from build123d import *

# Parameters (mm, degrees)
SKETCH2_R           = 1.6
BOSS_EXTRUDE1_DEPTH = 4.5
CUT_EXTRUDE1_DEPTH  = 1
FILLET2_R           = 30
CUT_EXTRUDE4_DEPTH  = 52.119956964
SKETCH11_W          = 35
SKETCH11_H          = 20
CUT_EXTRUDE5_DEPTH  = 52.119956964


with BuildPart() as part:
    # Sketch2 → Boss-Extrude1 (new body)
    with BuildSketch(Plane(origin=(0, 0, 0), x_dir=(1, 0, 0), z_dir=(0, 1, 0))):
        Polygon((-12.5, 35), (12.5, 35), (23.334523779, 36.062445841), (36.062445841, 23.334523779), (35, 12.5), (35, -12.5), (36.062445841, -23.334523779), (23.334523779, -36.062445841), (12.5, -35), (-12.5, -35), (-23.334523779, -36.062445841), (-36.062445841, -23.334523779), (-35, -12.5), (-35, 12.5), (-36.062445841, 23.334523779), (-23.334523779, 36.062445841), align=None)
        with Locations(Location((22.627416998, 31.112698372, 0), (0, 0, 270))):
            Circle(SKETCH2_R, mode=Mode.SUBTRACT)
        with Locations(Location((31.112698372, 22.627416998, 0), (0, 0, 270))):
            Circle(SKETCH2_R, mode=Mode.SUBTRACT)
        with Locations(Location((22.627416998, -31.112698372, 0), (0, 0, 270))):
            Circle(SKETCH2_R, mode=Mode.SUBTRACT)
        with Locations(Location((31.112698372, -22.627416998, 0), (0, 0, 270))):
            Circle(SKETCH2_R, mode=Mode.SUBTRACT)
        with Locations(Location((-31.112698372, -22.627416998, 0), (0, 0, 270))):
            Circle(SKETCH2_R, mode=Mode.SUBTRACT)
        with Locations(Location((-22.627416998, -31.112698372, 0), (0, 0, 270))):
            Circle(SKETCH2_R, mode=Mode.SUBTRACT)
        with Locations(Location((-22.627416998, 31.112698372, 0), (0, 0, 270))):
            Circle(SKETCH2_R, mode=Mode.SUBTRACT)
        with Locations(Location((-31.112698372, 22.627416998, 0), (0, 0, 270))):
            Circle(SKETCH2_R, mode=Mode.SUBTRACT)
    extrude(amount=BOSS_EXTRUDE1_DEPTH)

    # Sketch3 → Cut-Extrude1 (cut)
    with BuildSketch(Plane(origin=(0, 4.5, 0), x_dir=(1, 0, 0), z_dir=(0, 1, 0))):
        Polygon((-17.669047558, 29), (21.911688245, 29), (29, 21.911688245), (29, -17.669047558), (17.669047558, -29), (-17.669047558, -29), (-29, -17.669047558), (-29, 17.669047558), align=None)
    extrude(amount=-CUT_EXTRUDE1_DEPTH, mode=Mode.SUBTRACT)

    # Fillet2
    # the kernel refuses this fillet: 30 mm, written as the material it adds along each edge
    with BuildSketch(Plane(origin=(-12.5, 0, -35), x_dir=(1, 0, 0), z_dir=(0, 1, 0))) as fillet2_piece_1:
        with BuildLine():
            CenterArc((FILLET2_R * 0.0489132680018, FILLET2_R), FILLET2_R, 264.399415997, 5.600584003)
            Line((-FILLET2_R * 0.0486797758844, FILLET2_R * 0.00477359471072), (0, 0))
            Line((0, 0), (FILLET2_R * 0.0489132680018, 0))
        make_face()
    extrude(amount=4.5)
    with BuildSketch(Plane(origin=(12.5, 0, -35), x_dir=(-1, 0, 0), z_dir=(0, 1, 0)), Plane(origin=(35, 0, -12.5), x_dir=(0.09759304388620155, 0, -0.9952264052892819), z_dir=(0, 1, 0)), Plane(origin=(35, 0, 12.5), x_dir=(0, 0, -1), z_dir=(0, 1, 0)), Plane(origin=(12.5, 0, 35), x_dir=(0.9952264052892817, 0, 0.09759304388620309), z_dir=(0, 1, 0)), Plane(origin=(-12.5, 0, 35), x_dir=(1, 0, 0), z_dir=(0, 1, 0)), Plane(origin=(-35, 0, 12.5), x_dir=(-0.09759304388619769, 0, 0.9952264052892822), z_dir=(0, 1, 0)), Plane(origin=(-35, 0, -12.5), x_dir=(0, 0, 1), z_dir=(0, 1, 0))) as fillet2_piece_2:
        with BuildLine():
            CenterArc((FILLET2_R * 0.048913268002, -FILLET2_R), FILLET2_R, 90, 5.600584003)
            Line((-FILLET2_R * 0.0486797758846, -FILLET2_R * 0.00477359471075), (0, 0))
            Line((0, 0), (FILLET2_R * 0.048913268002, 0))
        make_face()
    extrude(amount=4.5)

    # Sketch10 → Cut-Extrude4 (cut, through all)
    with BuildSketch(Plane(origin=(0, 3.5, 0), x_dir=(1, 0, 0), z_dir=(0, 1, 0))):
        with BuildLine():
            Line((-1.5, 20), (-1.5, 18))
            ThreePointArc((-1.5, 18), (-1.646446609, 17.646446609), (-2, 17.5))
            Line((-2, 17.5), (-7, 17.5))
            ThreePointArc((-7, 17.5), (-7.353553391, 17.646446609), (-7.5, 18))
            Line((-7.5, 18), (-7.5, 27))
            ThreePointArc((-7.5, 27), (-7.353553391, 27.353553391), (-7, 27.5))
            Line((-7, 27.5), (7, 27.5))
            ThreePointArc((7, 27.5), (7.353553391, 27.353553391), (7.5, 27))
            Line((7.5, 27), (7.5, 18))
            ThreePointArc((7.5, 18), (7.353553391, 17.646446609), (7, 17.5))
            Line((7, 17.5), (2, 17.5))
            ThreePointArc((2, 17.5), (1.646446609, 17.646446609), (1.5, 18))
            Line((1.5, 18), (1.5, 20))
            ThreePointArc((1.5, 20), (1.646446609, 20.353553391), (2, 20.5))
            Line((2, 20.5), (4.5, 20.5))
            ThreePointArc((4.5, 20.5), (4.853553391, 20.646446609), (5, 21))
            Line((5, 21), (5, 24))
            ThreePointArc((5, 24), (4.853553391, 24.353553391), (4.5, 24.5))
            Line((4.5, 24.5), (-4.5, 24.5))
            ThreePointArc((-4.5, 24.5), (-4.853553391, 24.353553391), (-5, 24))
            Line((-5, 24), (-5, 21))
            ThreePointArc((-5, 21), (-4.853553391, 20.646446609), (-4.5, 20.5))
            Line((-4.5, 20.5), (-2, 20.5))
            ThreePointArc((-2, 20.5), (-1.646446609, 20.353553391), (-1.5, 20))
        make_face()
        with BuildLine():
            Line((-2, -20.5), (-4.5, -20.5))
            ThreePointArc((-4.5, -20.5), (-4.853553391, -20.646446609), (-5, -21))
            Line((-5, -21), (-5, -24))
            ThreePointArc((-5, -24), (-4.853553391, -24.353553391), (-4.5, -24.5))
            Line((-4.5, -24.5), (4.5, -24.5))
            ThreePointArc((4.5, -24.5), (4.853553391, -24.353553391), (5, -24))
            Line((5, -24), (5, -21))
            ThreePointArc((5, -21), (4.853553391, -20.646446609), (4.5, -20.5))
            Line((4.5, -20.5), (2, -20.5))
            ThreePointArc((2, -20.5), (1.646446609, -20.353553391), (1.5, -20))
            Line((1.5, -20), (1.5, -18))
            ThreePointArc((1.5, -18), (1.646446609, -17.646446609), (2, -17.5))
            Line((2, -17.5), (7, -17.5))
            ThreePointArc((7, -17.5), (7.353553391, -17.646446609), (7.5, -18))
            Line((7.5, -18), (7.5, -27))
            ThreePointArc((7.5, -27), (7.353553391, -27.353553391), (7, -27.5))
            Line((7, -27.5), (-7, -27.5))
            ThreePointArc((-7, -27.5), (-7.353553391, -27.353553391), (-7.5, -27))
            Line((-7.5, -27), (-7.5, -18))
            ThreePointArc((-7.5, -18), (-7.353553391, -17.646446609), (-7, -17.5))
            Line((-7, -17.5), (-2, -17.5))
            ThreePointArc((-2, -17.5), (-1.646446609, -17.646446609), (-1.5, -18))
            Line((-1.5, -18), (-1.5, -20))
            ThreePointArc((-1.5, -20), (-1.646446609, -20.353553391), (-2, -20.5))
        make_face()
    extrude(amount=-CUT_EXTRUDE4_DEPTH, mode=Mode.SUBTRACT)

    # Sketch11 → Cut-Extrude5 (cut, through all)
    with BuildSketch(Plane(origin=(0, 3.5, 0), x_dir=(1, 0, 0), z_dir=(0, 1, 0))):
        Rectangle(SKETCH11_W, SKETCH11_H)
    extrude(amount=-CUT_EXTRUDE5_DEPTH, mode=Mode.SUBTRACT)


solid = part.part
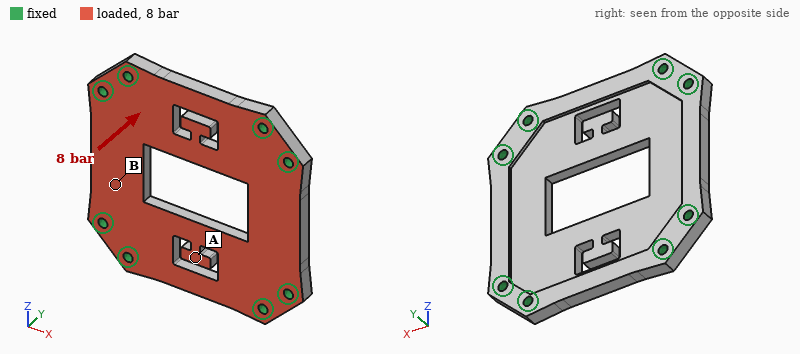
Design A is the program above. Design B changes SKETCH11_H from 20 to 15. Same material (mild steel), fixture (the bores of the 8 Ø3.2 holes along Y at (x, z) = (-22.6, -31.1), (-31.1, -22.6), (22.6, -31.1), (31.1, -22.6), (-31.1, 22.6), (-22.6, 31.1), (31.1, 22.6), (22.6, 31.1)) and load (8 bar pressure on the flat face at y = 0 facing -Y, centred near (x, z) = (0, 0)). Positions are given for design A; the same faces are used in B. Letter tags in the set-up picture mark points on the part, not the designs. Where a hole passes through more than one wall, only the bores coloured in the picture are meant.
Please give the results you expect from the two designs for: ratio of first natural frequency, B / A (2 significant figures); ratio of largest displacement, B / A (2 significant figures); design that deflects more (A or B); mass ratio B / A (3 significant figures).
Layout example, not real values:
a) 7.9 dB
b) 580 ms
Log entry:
a) 0.91
b) 1.2
c) B
d) 1.04
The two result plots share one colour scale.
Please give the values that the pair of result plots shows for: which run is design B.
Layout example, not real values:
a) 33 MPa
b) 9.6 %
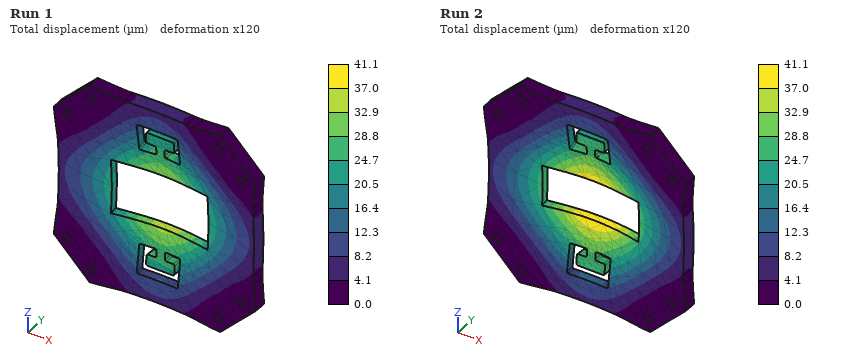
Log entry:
a) Run 2
